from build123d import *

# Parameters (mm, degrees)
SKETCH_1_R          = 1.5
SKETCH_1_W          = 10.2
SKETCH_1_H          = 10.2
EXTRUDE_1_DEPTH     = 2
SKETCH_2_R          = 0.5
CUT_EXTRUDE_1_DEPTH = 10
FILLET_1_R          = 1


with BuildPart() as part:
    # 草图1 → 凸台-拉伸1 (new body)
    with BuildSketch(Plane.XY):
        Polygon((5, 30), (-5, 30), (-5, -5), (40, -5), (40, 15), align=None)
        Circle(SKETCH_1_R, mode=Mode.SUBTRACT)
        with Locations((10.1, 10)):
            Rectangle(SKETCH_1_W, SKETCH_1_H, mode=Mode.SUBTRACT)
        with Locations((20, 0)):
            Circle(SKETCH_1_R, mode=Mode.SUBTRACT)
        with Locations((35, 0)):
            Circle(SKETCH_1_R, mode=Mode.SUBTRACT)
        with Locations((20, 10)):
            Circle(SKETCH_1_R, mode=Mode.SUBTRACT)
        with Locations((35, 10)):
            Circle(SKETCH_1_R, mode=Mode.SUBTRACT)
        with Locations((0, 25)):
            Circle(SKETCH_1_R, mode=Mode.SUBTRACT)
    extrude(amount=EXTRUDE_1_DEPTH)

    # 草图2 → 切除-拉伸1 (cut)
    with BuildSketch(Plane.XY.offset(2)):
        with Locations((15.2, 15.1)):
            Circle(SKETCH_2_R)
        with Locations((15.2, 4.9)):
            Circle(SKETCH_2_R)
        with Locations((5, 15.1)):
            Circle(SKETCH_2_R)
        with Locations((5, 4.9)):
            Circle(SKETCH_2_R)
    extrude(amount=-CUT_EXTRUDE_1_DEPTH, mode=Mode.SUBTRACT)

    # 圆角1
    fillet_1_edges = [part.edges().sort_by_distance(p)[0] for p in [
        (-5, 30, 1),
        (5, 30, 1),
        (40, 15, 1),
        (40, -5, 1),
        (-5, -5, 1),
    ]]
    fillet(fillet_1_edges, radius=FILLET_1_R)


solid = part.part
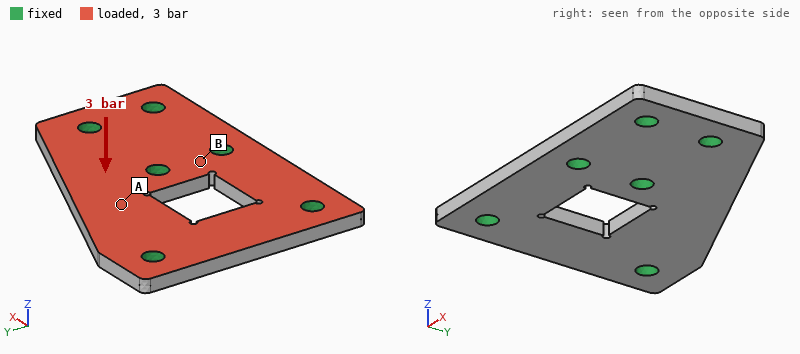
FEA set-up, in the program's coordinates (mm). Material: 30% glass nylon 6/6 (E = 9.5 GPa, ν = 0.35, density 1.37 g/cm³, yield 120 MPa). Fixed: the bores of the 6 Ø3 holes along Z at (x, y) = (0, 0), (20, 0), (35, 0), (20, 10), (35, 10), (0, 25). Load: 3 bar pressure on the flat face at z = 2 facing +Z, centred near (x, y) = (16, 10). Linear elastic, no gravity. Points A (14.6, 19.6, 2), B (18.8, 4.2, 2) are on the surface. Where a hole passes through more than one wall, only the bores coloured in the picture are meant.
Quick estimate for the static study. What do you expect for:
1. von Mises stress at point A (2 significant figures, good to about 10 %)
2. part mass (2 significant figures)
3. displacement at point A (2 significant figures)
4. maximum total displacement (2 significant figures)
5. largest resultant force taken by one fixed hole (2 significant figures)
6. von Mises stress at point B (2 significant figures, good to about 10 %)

12 MPa
3.2 g
0.068 mm
0.11 mm
80 N
4.2 MPa
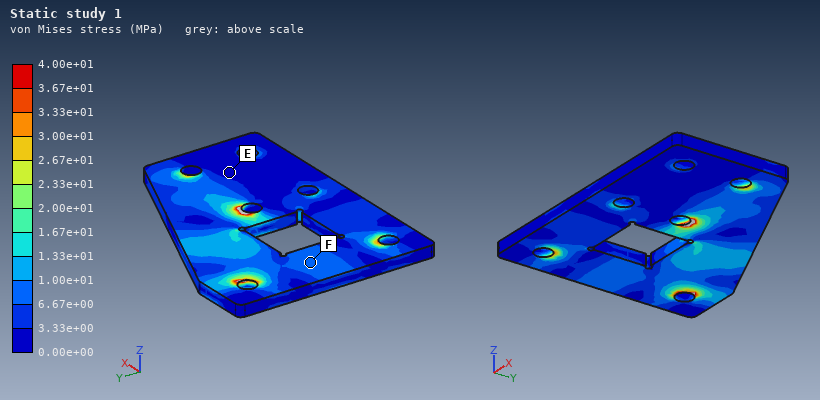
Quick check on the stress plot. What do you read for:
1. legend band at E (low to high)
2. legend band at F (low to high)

0.00e+00 to 3.33e+00 MPa
6.67e+00 to 1.00e+01 MPa
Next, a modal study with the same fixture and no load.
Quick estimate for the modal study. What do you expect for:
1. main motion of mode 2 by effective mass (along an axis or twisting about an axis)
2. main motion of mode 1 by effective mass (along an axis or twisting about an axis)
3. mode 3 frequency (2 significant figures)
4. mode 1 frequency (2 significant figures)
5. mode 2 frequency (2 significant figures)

along Z
along Z
11 kHz
6500 Hz
9200 Hz
